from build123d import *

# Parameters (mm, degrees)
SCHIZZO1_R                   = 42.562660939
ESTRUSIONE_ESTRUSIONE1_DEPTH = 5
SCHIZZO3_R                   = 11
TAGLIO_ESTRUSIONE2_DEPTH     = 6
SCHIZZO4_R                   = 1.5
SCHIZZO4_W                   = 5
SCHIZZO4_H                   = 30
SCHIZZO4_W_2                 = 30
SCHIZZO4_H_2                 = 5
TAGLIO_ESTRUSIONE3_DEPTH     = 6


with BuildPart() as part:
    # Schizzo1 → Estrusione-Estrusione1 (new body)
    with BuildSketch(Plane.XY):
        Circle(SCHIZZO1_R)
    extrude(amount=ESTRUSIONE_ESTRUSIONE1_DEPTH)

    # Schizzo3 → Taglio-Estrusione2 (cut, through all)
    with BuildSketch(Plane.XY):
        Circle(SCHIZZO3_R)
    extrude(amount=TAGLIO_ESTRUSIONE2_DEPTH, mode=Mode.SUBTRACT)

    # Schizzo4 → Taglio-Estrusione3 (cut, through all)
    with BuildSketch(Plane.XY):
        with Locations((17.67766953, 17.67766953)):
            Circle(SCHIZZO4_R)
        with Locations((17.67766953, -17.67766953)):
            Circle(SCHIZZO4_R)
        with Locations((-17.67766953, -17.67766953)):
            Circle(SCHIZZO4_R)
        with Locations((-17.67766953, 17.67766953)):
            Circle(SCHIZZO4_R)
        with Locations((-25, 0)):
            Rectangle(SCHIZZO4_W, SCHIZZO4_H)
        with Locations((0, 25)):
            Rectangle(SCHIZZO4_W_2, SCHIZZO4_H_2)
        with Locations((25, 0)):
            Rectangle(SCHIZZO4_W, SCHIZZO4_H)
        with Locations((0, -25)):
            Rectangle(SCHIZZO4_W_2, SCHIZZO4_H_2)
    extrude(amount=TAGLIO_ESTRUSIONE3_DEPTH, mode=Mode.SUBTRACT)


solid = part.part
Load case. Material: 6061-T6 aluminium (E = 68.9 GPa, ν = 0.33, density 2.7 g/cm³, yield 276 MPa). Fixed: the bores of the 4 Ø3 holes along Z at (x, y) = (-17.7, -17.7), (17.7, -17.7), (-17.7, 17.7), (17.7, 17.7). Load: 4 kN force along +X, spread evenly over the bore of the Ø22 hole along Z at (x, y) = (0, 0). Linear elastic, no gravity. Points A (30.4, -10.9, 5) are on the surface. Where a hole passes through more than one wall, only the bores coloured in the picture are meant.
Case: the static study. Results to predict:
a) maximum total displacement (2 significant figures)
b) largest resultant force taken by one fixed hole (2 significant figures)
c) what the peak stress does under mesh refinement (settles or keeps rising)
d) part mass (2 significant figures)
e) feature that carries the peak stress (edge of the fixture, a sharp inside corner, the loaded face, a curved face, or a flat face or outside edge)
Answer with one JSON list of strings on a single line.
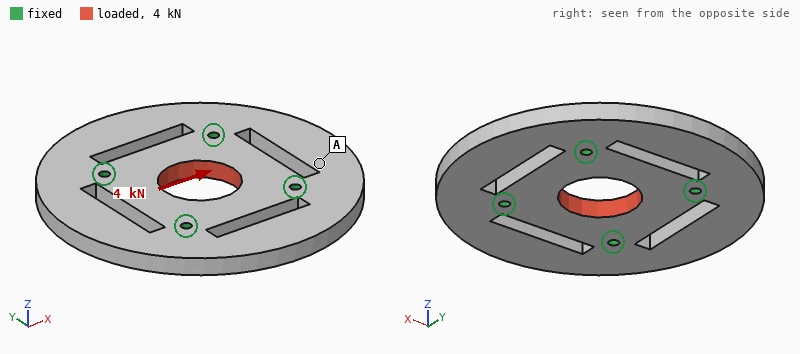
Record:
["7.8 µm", "1.1 kN", "keeps rising", "63 g", "edge of the fixture"]
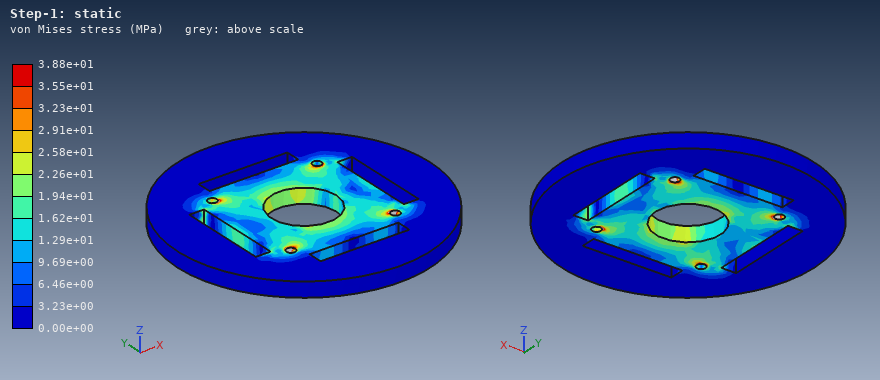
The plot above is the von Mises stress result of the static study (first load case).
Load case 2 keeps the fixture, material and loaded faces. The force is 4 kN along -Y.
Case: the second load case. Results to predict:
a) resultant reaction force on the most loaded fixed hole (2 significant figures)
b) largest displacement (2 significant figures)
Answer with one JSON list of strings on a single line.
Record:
["1.1 kN", "7.7 µm"]
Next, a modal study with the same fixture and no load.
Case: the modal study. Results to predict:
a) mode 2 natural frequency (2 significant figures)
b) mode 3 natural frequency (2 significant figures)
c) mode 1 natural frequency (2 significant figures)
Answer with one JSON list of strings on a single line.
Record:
["5400 Hz", "5400 Hz", "4600 Hz"]
